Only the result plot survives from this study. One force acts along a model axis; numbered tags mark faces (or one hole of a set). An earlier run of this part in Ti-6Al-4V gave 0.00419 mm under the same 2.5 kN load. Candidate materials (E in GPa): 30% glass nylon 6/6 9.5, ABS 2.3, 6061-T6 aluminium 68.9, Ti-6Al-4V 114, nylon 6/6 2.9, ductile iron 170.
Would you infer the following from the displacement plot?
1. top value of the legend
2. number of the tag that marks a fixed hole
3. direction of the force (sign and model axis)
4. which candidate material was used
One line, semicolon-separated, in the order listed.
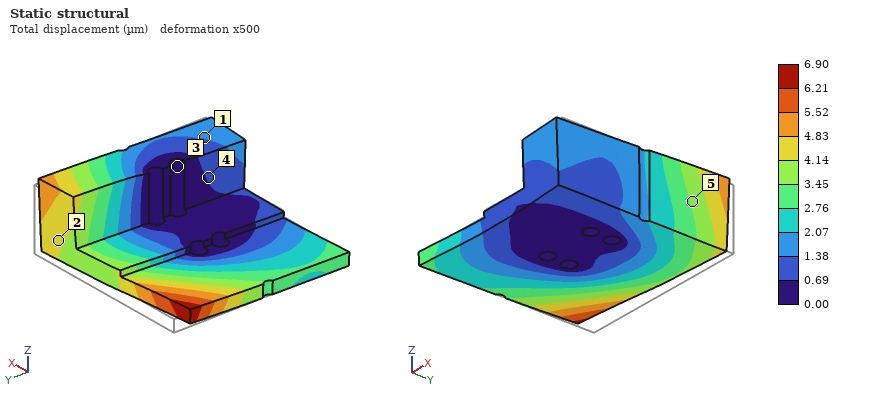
6.90 µm; 3; -Y; 6061-T6 aluminium
